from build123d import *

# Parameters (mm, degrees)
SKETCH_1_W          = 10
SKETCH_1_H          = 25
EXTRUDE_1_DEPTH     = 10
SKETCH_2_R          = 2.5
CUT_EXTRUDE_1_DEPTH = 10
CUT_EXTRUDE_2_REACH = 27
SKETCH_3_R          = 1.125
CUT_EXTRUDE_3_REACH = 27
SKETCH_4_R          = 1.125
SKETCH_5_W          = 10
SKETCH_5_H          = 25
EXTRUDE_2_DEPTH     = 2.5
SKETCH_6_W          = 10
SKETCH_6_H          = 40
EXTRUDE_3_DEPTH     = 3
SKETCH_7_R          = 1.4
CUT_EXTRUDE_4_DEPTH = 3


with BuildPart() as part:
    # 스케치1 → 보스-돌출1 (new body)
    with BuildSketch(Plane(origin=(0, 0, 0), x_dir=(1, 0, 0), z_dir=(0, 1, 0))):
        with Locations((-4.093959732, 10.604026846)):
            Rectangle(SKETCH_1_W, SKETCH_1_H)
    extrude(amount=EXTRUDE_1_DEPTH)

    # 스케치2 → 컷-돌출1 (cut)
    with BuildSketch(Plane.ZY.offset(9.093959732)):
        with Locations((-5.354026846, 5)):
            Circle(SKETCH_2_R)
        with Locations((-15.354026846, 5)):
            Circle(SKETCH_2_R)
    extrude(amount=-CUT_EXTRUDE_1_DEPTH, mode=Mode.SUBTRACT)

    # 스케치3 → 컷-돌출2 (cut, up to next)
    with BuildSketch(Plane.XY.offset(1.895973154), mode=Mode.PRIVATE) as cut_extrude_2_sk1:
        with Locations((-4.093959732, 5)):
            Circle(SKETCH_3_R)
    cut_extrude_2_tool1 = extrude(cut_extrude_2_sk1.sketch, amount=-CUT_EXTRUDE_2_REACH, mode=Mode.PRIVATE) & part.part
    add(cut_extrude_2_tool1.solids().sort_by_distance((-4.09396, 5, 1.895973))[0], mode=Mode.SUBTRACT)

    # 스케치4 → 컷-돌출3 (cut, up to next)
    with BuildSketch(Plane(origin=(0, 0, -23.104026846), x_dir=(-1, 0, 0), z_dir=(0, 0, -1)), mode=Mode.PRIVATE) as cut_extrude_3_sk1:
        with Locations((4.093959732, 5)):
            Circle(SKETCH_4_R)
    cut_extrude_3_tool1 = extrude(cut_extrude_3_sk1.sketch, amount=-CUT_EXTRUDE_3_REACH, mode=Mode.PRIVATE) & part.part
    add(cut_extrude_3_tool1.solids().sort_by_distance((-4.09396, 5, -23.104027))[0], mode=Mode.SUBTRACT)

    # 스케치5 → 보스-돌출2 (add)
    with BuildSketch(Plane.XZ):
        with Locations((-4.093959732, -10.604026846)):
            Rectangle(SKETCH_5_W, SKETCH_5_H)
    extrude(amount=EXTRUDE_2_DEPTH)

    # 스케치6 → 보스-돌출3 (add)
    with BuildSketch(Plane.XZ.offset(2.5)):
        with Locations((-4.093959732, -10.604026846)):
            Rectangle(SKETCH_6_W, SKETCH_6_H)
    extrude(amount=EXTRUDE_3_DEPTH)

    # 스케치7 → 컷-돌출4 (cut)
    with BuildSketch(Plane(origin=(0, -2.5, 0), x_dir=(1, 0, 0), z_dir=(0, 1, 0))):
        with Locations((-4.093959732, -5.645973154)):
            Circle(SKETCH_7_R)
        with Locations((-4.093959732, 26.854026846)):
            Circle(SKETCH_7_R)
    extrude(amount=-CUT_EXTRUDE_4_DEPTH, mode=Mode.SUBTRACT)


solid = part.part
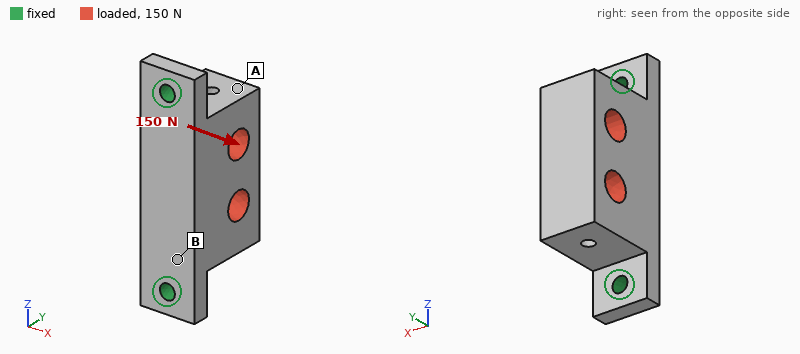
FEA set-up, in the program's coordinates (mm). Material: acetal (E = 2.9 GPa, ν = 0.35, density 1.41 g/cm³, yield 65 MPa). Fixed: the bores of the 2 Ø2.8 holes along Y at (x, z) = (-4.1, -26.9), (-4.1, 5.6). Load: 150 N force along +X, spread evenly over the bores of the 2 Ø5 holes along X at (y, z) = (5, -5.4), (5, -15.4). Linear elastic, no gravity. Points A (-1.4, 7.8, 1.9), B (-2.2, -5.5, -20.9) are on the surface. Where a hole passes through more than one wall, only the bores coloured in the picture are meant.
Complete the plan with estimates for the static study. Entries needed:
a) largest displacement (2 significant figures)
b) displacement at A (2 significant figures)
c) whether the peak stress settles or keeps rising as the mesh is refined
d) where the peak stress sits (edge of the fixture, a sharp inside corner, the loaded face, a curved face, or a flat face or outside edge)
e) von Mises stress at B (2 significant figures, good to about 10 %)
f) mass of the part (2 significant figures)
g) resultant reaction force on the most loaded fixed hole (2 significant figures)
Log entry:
0.47 mm
0.38 mm
keeps rising
edge of the fixture
9.3 MPa
5.4 g
76 N
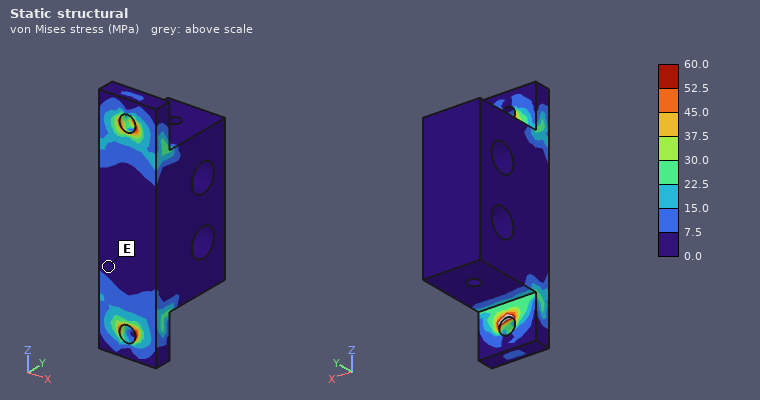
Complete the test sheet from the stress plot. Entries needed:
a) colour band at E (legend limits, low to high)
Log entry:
0.0 to 7.5 MPa
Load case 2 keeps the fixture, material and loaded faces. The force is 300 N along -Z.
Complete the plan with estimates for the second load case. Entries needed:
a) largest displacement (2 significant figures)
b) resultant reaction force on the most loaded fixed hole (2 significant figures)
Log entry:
65 µm
180 N
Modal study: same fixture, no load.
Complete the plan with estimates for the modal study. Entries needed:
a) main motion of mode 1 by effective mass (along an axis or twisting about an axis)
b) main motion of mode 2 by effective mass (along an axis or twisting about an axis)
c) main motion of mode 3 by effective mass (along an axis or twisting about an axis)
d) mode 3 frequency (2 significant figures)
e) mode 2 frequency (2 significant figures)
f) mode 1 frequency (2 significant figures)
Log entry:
along X
along Y
along Z
6500 Hz
5000 Hz
1900 Hz
